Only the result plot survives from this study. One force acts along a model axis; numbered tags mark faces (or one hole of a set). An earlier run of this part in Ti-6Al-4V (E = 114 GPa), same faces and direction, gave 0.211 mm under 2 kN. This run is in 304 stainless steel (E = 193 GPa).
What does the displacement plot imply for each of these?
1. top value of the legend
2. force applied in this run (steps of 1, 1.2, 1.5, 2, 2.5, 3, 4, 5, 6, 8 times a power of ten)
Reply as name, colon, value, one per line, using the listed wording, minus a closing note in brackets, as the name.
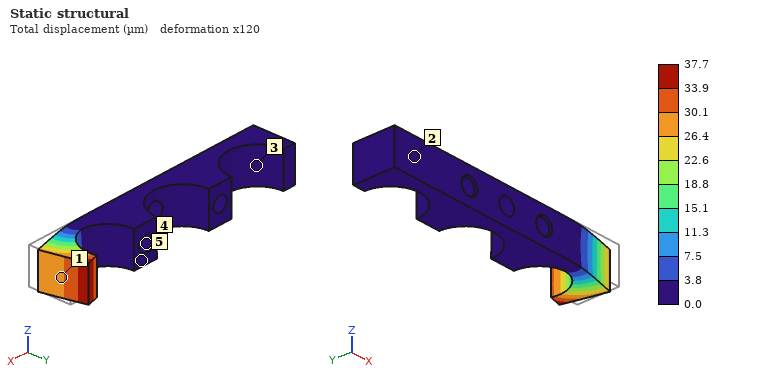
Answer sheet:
top value of the legend: 37.7 µm
force applied in this run: 600 N
